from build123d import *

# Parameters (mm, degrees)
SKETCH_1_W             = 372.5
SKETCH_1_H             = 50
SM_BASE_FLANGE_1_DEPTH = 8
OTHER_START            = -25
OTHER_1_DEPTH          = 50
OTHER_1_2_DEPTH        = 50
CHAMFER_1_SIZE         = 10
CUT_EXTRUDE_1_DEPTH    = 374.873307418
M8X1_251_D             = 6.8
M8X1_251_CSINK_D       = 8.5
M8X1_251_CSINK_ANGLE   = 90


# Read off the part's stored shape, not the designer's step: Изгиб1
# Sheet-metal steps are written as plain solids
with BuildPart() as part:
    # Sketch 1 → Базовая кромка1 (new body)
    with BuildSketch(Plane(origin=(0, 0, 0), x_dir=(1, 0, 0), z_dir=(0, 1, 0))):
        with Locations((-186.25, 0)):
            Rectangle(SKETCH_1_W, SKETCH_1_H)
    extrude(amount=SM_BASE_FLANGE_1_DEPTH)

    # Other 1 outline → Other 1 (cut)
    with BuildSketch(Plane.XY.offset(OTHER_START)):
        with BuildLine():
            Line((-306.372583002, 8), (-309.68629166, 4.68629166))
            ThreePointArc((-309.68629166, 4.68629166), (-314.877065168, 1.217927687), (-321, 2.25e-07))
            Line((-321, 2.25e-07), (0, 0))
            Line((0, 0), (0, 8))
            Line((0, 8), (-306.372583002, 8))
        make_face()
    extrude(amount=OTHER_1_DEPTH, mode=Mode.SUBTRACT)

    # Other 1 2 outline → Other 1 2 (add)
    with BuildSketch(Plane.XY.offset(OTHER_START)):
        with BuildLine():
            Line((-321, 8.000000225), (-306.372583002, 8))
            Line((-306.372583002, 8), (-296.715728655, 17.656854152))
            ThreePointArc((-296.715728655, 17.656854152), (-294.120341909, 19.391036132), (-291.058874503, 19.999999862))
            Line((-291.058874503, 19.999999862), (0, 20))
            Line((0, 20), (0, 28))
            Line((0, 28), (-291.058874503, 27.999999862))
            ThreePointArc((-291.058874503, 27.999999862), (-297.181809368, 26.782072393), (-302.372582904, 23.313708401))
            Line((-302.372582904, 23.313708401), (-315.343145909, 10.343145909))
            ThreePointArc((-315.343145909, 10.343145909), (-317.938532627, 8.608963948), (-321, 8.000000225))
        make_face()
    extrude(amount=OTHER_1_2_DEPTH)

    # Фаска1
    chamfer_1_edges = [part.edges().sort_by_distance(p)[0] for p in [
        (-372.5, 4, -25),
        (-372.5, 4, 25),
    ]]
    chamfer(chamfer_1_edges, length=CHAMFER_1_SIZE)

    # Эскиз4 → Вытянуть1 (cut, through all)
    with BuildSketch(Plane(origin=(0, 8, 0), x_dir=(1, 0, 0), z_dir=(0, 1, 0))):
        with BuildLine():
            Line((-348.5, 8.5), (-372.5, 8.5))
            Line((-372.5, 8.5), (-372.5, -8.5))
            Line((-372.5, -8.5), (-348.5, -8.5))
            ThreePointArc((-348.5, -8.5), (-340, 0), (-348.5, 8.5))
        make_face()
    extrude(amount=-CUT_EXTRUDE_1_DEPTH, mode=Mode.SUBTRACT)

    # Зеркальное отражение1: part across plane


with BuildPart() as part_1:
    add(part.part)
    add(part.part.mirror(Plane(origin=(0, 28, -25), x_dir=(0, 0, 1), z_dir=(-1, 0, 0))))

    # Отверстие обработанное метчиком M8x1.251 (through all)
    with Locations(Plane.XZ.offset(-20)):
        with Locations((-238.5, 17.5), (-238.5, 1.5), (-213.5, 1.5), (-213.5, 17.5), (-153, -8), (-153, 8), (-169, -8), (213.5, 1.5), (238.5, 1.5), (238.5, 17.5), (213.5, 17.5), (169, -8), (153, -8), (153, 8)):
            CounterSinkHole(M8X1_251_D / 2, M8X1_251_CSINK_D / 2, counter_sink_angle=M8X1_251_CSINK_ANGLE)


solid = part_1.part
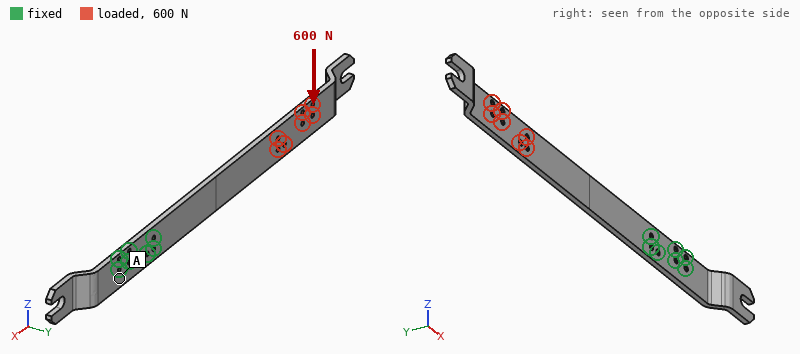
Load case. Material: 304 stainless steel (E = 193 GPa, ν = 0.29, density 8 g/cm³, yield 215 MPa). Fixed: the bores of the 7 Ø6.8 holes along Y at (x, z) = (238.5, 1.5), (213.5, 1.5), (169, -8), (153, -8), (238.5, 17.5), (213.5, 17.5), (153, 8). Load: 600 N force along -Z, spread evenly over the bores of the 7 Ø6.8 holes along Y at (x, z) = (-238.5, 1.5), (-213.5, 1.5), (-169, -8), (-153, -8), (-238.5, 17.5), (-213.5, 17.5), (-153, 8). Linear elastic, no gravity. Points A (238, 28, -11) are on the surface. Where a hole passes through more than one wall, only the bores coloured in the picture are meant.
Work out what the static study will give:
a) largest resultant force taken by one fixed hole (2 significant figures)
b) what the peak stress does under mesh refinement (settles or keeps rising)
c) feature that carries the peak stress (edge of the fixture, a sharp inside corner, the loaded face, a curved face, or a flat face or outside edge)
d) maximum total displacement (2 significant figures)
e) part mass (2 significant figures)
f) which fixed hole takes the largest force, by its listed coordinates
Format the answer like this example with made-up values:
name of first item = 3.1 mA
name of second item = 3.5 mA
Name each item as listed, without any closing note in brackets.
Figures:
largest resultant force taken by one fixed hole = 6.2 kN
what the peak stress does under mesh refinement = keeps rising
feature that carries the peak stress = edge of the fixture
maximum total displacement = 1.0 mm
part mass = 2.3 kg
which fixed hole takes the largest force, by its listed coordinates = (153, 8)
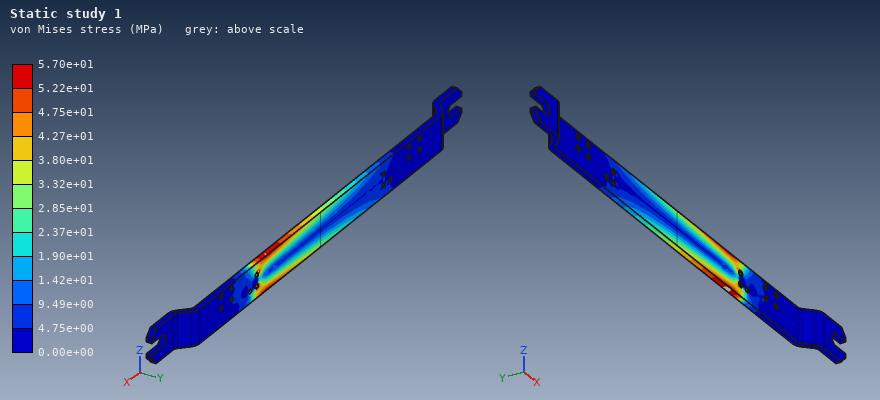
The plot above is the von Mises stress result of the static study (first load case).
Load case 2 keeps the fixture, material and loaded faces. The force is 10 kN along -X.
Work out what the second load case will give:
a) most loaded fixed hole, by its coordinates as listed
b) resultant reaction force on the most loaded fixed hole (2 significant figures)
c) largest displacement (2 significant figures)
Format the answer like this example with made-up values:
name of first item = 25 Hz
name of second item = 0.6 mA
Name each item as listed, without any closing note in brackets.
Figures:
most loaded fixed hole, by its coordinates as listed = (153, 8)
resultant reaction force on the most loaded fixed hole = 5.8 kN
largest displacement = 1.3 mm
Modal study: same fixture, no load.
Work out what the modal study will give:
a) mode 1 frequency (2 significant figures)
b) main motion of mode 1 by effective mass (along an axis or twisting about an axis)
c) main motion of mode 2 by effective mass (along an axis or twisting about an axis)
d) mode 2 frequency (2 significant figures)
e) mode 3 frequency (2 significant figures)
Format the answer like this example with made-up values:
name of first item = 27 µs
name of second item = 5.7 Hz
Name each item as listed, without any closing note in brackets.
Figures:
mode 1 frequency = 24 Hz
main motion of mode 1 by effective mass = along Y
main motion of mode 2 by effective mass = along Z
mode 2 frequency = 140 Hz
mode 3 frequency = 150 Hz
